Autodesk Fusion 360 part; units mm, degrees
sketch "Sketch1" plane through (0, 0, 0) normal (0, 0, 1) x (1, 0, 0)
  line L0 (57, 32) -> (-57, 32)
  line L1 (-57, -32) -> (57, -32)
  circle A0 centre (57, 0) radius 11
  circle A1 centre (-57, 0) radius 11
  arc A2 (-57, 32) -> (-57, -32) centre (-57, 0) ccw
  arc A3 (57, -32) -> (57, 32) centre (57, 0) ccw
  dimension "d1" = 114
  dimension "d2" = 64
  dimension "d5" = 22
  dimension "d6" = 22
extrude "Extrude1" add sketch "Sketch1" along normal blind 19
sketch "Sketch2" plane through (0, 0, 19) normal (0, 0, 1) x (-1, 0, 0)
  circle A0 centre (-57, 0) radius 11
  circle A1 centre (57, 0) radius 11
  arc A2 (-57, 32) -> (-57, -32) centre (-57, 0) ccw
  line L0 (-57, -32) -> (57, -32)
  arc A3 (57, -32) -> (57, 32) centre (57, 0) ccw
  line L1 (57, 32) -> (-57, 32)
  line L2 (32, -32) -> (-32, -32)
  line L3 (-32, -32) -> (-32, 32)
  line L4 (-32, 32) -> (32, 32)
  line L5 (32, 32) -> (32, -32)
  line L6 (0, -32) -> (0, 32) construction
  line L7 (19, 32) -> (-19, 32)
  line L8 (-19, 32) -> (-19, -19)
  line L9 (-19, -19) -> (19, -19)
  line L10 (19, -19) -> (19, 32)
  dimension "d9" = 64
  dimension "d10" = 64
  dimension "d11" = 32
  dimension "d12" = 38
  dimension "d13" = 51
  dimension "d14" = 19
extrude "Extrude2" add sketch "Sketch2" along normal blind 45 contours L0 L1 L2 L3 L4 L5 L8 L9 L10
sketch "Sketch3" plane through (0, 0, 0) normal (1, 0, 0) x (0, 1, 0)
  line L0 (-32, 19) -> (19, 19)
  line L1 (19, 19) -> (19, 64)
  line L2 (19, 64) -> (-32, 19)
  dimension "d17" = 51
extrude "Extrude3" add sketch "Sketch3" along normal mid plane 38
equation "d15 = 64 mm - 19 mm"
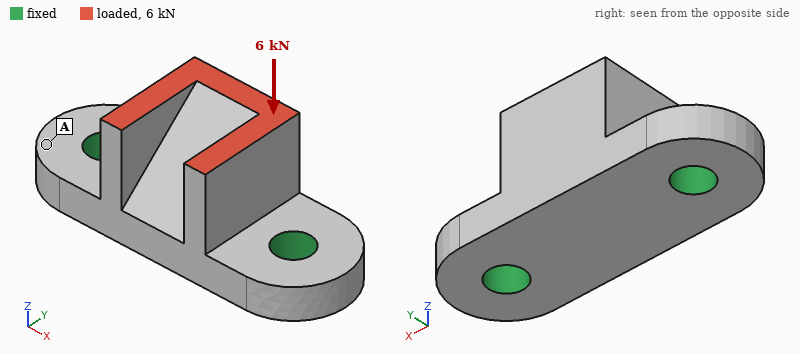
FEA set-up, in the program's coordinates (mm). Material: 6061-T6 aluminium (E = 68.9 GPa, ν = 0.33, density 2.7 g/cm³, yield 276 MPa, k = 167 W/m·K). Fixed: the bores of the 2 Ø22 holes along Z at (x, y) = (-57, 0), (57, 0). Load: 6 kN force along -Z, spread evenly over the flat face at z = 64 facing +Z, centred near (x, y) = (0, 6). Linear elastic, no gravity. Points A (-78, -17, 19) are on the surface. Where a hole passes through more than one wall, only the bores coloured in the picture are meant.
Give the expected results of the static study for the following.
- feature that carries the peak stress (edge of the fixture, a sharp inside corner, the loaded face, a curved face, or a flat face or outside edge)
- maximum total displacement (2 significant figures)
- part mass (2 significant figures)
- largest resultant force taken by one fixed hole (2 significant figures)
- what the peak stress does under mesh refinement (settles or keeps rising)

edge of the fixture
13 µm
880 g
3.2 kN
keeps rising
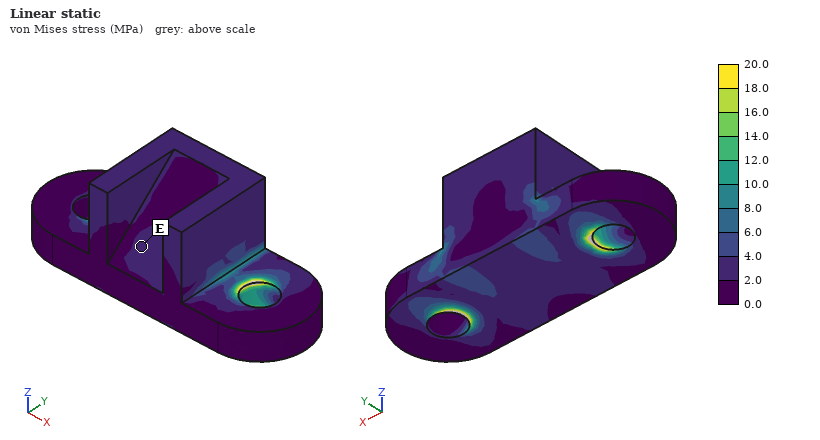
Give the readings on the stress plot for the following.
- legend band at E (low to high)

2.0 to 4.0 MPa
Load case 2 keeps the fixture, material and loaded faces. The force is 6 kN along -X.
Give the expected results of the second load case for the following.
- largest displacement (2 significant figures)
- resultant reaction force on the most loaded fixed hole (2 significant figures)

43 µm
4.9 kN
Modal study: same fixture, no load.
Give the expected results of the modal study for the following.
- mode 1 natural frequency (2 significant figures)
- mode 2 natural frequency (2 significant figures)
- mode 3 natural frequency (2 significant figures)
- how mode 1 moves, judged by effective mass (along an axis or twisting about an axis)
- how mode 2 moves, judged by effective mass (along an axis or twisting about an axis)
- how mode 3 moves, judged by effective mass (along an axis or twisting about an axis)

3500 Hz
6300 Hz
7100 Hz
along Y
along Z
along X
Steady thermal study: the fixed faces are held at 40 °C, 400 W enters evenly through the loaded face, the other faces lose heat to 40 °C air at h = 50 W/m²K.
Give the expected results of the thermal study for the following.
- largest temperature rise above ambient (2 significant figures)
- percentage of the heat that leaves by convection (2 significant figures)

68 K
12 %
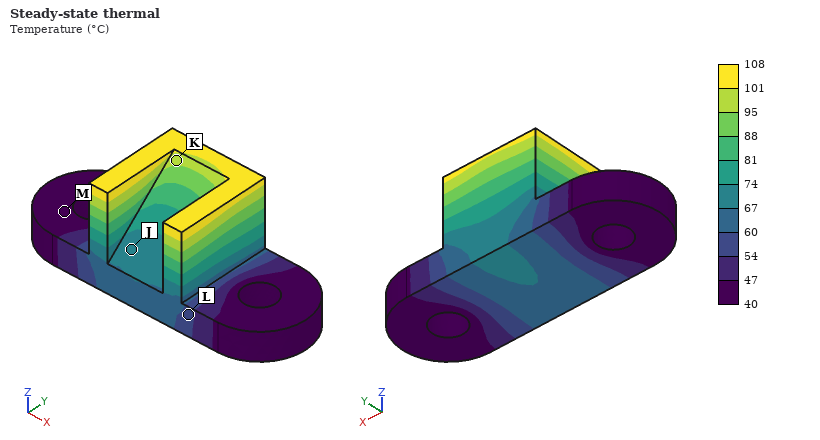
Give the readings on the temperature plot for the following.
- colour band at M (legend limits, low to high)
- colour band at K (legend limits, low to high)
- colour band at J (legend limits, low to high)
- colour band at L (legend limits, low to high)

40 to 47 °C
95 to 101 °C
67 to 74 °C
54 to 60 °C
